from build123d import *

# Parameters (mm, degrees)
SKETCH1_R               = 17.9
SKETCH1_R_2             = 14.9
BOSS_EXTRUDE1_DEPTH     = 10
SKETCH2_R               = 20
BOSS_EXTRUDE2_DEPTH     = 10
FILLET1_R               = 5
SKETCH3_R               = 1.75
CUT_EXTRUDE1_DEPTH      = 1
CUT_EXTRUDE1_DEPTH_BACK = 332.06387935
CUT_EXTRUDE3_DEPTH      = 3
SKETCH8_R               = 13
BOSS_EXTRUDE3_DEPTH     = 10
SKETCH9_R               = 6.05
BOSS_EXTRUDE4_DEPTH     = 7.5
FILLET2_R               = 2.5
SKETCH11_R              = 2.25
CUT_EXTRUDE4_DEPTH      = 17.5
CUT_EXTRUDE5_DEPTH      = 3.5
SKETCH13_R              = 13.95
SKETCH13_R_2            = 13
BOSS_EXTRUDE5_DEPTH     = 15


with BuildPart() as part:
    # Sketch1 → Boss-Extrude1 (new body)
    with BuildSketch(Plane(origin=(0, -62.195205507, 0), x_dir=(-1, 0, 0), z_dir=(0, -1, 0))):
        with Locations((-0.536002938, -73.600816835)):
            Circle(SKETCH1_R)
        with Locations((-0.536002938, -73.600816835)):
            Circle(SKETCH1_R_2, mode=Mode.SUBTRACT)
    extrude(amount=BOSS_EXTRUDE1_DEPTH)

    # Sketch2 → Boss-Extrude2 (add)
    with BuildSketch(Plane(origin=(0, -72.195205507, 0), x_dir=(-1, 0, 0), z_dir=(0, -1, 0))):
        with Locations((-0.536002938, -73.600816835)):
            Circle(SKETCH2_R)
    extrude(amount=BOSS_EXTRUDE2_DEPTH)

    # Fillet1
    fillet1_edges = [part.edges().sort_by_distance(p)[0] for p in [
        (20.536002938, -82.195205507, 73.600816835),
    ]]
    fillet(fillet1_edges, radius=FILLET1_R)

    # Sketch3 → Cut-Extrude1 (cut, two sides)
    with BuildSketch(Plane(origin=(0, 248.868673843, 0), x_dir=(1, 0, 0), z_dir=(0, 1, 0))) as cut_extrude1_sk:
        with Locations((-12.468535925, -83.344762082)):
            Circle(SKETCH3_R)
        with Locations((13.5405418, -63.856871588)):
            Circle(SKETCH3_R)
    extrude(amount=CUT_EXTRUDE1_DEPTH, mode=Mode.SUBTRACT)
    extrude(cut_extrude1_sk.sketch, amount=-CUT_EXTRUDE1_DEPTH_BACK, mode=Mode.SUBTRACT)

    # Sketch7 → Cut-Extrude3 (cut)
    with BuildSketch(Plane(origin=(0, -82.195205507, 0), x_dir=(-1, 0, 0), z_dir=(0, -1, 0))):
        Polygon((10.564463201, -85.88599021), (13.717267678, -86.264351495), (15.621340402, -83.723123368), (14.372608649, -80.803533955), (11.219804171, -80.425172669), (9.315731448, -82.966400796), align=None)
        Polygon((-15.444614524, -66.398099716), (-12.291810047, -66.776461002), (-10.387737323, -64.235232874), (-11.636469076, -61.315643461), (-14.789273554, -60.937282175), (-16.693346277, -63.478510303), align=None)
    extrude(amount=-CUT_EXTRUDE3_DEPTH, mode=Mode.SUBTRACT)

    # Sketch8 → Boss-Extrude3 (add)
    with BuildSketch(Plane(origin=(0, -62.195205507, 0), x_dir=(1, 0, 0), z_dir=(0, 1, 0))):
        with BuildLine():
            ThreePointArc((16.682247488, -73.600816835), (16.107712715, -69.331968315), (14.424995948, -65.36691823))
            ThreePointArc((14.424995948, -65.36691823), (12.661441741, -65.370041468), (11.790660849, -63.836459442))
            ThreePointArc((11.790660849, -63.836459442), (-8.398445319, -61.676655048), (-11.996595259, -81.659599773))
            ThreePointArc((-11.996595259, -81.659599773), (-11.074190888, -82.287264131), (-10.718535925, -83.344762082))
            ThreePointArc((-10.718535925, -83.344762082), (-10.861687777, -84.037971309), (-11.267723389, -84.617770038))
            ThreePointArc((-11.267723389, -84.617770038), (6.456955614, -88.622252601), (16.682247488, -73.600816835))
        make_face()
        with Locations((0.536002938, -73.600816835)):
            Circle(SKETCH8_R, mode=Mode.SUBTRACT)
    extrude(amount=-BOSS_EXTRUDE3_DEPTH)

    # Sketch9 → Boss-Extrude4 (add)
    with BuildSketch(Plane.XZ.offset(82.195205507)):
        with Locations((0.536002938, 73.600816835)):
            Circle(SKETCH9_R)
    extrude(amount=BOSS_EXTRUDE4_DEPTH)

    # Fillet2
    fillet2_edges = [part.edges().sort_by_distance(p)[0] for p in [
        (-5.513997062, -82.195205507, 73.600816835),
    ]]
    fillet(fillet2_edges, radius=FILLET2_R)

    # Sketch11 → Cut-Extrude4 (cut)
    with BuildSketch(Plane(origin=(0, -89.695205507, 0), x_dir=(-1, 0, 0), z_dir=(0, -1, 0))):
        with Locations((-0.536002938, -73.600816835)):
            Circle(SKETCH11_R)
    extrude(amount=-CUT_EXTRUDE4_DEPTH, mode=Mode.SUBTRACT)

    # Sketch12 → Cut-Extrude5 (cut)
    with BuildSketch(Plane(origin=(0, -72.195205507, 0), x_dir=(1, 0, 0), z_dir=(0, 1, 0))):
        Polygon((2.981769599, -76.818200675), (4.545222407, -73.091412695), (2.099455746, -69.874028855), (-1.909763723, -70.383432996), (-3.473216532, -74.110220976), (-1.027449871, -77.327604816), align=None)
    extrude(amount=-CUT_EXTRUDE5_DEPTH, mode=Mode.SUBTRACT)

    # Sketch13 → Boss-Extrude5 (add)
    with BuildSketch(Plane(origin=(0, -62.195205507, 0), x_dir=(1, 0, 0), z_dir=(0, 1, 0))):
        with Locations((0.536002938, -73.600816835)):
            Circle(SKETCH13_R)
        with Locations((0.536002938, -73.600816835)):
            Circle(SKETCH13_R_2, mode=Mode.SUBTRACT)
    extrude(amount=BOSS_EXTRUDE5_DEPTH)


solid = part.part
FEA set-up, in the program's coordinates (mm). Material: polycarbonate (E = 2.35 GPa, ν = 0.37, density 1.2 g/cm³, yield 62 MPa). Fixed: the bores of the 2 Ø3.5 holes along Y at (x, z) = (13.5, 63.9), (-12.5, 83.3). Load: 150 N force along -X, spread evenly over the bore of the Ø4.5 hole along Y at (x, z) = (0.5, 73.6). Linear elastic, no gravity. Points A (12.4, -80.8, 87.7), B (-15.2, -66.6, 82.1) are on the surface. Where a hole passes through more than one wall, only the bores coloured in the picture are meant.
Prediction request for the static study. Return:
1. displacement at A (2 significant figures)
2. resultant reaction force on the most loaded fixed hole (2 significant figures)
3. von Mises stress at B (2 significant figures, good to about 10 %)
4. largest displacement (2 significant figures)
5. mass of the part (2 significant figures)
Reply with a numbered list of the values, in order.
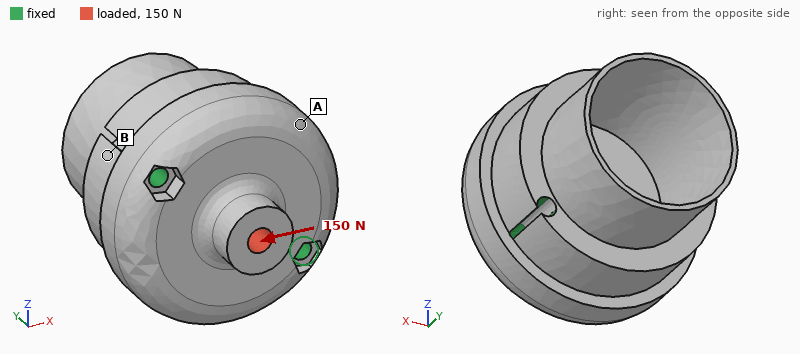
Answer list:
1. 8.8 µm
2. 81 N
3. 0.55 MPa
4. 19 µm
5. 22 g
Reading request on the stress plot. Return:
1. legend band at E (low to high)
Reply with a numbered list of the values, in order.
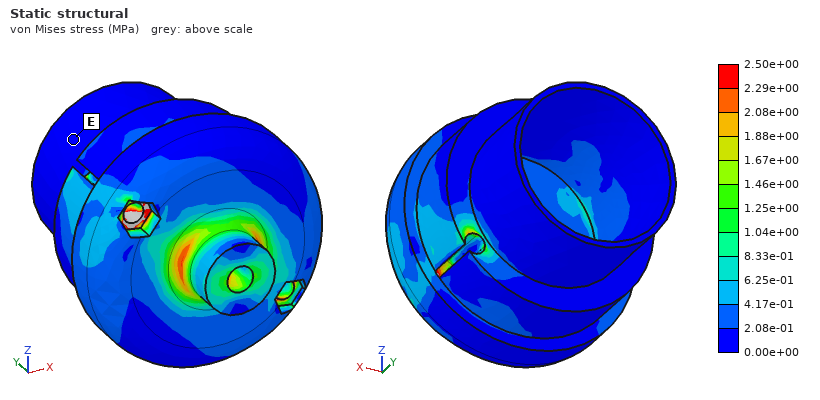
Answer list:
1. 0.00e+00 to 2.08e-01 MPa
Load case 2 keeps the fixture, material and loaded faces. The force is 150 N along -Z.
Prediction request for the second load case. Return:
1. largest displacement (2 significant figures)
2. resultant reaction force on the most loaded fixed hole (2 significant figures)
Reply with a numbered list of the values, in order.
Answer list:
1. 22 µm
2. 78 N
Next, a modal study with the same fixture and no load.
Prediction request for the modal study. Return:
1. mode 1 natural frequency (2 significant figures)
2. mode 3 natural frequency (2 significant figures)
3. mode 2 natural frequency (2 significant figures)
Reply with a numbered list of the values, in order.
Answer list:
1. 4300 Hz
2. 4600 Hz
3. 4400 Hz
